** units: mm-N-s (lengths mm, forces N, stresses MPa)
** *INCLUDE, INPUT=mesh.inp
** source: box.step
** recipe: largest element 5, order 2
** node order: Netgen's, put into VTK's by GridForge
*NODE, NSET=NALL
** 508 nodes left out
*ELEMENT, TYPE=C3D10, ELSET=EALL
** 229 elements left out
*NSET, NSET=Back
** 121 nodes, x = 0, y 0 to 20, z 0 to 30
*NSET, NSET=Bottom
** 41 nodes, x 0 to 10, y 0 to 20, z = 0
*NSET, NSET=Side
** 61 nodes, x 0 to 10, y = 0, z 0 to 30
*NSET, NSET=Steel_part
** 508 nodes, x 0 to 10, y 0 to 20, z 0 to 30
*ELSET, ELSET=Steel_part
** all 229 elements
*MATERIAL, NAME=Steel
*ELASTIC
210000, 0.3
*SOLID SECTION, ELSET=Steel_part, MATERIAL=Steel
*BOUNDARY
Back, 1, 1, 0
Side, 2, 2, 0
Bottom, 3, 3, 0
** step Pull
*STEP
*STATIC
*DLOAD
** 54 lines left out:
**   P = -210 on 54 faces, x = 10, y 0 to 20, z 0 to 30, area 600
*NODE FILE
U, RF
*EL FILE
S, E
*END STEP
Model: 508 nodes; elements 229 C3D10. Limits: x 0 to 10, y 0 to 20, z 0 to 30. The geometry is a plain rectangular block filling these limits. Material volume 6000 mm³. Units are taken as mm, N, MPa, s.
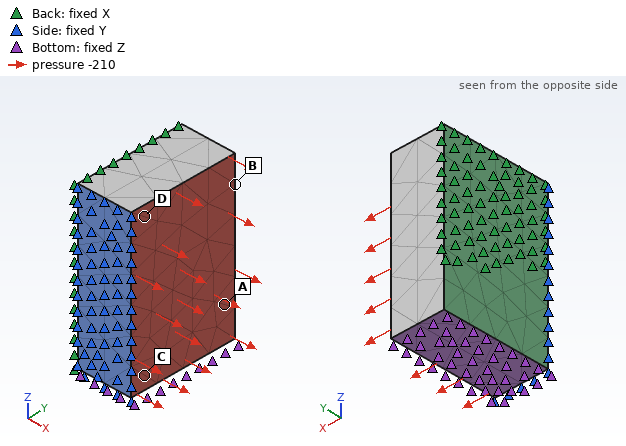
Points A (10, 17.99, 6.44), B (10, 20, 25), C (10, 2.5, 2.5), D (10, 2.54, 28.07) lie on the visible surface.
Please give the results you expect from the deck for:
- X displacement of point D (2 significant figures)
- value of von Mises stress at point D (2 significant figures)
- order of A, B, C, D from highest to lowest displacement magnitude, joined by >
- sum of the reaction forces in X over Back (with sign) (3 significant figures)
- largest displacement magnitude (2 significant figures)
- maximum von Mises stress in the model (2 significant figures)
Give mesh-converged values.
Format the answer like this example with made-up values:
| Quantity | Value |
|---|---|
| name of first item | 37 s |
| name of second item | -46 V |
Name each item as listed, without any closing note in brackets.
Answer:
| Quantity | Value |
|---|---|
| X displacement of point D | 0.010 mm |
| value of von Mises stress at point D | 210 MPa |
| order of A, B, C, D from highest to lowest displacement magnitude, joined by > | B > D > A > C |
| sum of the reaction forces in X over Back (with sign) | -1.26e+05 N |
| largest displacement magnitude | 0.015 mm |
| maximum von Mises stress in the model | 210 MPa |
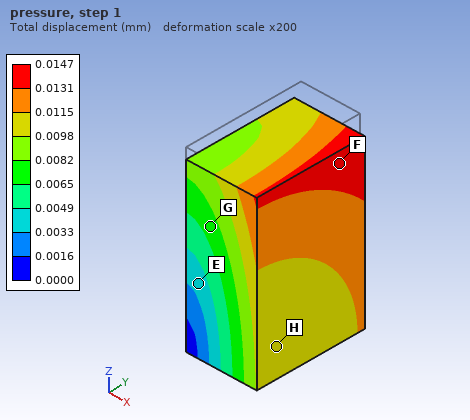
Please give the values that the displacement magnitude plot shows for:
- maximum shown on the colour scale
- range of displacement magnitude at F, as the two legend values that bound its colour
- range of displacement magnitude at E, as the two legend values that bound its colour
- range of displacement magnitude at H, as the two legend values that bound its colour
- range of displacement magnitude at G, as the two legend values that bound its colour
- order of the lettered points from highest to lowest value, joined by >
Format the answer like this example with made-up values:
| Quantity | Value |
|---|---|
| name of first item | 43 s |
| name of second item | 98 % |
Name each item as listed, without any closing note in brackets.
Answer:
| Quantity | Value |
|---|---|
| maximum shown on the colour scale | 0.0147 mm |
| range of displacement magnitude at F, as the two legend values that bound its colour | 0.0131 to 0.0147 mm |
| range of displacement magnitude at E, as the two legend values that bound its colour | 0.0033 to 0.0049 mm |
| range of displacement magnitude at H, as the two legend values that bound its colour | 0.0098 to 0.0115 mm |
| range of displacement magnitude at G, as the two legend values that bound its colour | 0.0065 to 0.0082 mm |
| order of the lettered points from highest to lowest value, joined by > | F > H > G > E |
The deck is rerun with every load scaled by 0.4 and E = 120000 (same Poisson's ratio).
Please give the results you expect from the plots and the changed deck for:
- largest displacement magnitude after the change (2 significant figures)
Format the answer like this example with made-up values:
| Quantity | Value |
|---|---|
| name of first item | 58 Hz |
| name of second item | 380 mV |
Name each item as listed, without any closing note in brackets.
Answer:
| Quantity | Value |
|---|---|
| largest displacement magnitude after the change | 0.010 mm |
